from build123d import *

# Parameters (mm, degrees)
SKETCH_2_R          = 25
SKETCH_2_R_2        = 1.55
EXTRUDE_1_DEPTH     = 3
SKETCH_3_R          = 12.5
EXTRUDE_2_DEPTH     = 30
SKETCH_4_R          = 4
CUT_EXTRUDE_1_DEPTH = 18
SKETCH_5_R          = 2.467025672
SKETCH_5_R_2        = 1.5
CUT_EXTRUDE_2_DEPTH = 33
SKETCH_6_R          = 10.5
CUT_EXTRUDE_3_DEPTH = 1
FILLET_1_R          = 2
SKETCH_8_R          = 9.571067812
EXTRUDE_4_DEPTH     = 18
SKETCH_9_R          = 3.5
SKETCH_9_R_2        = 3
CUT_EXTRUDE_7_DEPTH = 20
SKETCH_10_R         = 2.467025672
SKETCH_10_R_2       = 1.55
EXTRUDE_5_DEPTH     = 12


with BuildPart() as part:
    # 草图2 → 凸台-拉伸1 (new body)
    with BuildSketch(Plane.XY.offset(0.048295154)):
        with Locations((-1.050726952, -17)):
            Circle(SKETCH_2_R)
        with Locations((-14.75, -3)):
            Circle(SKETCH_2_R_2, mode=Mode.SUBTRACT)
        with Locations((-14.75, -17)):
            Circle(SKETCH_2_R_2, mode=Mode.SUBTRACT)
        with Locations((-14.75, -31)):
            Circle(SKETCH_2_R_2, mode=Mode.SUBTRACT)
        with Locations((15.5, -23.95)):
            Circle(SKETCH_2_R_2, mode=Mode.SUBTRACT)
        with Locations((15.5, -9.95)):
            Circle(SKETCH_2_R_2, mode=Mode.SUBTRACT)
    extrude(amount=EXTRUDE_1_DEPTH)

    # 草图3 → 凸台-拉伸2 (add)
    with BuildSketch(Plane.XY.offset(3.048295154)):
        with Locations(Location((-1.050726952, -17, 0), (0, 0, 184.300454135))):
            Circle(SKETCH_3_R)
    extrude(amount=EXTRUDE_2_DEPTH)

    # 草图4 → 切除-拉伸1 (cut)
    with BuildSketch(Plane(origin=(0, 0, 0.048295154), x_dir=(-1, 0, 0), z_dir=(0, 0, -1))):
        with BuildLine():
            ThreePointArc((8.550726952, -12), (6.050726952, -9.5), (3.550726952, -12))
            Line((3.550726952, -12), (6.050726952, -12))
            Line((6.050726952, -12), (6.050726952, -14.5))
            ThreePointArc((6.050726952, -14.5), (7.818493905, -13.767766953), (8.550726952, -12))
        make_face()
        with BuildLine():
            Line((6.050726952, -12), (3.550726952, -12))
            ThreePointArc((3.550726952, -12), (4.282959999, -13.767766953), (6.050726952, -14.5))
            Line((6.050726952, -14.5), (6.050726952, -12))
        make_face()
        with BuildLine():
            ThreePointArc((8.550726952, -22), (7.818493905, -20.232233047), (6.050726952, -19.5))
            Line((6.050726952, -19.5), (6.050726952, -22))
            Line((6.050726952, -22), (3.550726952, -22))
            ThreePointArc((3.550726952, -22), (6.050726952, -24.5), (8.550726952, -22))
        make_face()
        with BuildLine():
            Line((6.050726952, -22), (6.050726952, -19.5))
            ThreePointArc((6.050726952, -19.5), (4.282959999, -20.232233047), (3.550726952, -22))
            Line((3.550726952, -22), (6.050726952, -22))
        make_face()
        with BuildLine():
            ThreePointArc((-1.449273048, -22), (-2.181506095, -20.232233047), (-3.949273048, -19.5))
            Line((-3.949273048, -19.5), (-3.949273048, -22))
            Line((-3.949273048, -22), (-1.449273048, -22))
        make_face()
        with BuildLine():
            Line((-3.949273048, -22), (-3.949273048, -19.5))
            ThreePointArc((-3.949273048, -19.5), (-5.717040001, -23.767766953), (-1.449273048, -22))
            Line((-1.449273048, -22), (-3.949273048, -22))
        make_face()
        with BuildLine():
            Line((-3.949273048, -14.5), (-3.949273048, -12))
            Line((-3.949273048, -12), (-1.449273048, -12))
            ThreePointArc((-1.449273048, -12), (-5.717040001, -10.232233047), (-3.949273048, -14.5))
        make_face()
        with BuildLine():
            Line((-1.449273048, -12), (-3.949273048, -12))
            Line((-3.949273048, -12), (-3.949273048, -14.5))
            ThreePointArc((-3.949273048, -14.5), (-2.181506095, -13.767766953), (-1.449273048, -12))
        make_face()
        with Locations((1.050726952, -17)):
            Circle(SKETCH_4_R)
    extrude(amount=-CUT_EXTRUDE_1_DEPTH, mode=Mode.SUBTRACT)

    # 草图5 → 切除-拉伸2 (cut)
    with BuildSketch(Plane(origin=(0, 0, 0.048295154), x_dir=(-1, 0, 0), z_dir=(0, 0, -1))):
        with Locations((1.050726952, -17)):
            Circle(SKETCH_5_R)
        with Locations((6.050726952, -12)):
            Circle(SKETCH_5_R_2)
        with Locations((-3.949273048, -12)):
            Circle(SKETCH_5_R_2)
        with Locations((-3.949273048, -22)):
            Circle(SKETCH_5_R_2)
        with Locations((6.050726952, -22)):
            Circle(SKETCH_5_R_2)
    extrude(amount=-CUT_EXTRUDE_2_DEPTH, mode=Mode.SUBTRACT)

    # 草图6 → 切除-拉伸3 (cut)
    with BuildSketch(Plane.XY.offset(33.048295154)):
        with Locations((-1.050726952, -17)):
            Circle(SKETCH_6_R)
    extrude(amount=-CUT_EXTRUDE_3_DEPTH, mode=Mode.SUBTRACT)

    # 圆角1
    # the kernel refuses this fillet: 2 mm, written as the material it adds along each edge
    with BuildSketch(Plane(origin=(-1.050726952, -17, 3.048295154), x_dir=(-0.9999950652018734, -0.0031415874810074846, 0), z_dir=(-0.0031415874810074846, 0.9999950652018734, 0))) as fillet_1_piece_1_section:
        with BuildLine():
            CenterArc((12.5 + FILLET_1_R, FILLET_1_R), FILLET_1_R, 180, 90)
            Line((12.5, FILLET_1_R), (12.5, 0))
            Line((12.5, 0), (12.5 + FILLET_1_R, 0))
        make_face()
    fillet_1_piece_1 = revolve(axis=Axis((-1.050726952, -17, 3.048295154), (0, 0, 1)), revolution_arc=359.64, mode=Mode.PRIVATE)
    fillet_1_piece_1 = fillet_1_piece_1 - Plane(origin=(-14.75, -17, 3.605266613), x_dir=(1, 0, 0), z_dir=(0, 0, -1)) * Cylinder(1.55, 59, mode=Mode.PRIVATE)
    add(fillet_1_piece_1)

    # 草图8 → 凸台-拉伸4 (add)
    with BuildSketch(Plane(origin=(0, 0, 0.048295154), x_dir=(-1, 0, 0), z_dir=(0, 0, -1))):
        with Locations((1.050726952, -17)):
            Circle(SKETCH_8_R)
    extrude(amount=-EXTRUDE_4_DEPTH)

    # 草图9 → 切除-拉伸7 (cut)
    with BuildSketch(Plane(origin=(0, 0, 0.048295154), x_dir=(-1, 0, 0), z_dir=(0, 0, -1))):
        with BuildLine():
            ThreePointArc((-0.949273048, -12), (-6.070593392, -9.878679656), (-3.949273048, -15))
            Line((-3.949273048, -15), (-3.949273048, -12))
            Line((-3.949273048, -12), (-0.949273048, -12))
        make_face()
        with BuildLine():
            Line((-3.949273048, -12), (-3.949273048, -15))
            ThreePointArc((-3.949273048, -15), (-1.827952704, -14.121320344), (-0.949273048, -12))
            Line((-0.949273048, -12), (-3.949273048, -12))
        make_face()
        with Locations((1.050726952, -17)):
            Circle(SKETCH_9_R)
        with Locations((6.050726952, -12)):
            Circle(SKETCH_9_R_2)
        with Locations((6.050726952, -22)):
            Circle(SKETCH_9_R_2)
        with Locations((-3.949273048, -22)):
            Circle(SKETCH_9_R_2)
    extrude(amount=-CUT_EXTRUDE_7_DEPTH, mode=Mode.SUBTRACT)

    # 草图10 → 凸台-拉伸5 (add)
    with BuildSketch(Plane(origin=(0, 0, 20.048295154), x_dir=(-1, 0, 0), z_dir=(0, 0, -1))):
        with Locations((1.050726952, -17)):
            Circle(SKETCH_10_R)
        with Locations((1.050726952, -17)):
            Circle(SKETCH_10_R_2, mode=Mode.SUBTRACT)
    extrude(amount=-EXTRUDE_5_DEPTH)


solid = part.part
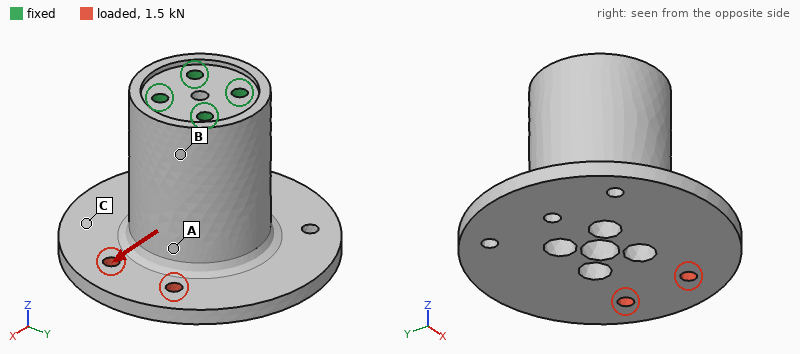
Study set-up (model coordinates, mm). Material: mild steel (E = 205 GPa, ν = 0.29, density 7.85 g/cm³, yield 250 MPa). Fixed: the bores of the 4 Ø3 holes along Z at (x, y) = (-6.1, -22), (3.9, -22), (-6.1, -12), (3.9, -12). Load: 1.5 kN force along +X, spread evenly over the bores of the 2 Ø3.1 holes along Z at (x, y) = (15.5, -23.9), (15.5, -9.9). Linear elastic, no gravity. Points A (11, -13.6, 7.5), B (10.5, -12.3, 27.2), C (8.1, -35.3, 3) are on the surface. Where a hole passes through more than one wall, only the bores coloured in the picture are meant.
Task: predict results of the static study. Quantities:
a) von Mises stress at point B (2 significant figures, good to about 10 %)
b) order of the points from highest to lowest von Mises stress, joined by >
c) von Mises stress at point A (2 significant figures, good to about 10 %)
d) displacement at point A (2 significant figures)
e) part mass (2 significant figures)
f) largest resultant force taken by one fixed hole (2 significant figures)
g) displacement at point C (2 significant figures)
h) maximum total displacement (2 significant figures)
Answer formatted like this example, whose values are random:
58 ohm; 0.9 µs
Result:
8.9 MPa; A > B > C; 13 MPa; 4.2 µm; 130 g; 1.0 kN; 4.7 µm; 9.7 µm
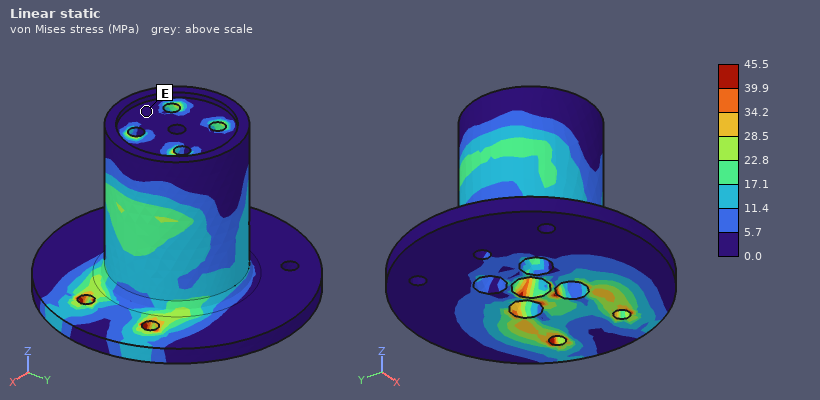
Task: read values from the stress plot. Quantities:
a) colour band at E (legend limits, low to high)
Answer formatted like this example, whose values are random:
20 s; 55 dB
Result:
0.0 to 5.7 MPa
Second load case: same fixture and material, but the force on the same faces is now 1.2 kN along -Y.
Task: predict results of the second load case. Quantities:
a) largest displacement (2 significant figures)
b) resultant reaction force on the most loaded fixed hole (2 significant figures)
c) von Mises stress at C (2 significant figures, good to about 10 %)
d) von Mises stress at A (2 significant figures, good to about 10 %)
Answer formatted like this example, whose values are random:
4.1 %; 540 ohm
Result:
10 µm; 1.2 kN; 5.6 MPa; 24 MPa
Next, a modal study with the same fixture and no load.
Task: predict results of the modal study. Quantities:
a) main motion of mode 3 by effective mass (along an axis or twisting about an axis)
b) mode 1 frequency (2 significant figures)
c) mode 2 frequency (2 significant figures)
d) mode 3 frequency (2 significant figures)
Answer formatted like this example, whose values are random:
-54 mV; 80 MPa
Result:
along Z; 9600 Hz; 9700 Hz; 12 kHz
